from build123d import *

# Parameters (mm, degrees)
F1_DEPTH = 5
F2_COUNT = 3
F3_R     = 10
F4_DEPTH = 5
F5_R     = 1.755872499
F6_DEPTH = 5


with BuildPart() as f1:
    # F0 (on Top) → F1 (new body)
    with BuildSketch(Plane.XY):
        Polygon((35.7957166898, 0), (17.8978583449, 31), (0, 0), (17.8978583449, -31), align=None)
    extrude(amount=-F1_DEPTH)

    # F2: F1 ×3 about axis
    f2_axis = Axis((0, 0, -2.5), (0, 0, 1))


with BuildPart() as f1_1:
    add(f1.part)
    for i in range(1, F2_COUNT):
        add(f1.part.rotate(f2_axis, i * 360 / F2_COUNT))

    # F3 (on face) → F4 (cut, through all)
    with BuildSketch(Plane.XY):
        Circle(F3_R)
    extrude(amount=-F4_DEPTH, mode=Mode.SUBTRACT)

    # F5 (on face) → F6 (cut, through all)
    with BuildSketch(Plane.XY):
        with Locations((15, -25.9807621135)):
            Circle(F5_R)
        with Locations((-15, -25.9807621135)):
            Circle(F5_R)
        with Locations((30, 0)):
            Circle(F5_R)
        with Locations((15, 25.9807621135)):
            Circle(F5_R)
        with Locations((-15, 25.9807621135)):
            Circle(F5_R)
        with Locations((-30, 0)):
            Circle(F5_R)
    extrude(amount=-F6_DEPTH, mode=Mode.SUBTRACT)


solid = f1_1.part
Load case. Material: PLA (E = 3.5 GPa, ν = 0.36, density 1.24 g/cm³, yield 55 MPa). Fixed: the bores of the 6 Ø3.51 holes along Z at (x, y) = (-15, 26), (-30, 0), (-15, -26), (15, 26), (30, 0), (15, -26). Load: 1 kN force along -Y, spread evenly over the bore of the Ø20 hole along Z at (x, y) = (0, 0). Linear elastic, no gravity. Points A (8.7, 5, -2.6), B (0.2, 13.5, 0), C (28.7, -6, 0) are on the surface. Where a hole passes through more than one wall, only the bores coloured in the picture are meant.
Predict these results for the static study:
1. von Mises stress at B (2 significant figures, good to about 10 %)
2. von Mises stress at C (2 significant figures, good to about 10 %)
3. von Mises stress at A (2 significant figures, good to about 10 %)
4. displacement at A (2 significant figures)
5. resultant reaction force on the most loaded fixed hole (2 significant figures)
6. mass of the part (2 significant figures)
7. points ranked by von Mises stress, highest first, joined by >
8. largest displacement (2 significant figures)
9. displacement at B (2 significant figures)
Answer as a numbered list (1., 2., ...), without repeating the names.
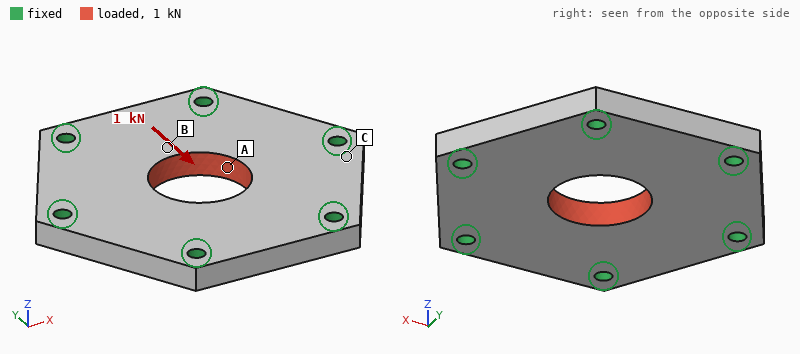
1. 2.7 MPa
2. 1.1 MPa
3. 4.9 MPa
4. 23 µm
5. 230 N
6. 18 g
7. A > B > C
8. 24 µm
9. 21 µm
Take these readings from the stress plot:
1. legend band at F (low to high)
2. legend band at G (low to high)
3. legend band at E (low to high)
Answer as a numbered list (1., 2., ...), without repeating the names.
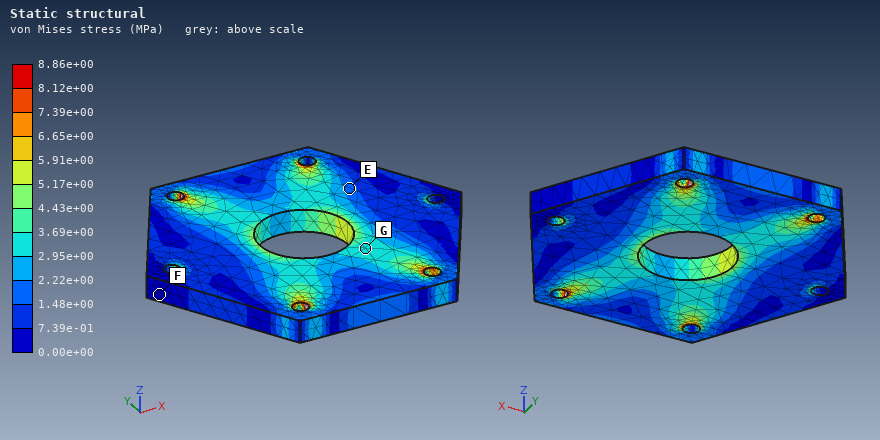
1. 0.00e+00 to 7.39e-01 MPa
2. 2.95e+00 to 3.69e+00 MPa
3. 1.48e+00 to 2.22e+00 MPa
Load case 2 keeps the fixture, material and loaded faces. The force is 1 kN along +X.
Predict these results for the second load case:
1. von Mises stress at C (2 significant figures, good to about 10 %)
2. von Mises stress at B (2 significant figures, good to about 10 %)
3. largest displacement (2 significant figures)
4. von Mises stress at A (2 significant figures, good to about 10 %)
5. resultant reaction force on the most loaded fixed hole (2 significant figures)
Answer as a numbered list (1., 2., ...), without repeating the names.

1. 1.7 MPa
2. 3.2 MPa
3. 23 µm
4. 3.7 MPa
5. 260 N
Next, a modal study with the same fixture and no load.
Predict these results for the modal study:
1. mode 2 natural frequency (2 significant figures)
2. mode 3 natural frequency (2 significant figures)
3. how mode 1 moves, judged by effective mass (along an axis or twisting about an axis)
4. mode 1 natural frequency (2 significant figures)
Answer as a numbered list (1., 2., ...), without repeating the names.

1. 6200 Hz
2. 6200 Hz
3. along Z
4. 3900 Hz
